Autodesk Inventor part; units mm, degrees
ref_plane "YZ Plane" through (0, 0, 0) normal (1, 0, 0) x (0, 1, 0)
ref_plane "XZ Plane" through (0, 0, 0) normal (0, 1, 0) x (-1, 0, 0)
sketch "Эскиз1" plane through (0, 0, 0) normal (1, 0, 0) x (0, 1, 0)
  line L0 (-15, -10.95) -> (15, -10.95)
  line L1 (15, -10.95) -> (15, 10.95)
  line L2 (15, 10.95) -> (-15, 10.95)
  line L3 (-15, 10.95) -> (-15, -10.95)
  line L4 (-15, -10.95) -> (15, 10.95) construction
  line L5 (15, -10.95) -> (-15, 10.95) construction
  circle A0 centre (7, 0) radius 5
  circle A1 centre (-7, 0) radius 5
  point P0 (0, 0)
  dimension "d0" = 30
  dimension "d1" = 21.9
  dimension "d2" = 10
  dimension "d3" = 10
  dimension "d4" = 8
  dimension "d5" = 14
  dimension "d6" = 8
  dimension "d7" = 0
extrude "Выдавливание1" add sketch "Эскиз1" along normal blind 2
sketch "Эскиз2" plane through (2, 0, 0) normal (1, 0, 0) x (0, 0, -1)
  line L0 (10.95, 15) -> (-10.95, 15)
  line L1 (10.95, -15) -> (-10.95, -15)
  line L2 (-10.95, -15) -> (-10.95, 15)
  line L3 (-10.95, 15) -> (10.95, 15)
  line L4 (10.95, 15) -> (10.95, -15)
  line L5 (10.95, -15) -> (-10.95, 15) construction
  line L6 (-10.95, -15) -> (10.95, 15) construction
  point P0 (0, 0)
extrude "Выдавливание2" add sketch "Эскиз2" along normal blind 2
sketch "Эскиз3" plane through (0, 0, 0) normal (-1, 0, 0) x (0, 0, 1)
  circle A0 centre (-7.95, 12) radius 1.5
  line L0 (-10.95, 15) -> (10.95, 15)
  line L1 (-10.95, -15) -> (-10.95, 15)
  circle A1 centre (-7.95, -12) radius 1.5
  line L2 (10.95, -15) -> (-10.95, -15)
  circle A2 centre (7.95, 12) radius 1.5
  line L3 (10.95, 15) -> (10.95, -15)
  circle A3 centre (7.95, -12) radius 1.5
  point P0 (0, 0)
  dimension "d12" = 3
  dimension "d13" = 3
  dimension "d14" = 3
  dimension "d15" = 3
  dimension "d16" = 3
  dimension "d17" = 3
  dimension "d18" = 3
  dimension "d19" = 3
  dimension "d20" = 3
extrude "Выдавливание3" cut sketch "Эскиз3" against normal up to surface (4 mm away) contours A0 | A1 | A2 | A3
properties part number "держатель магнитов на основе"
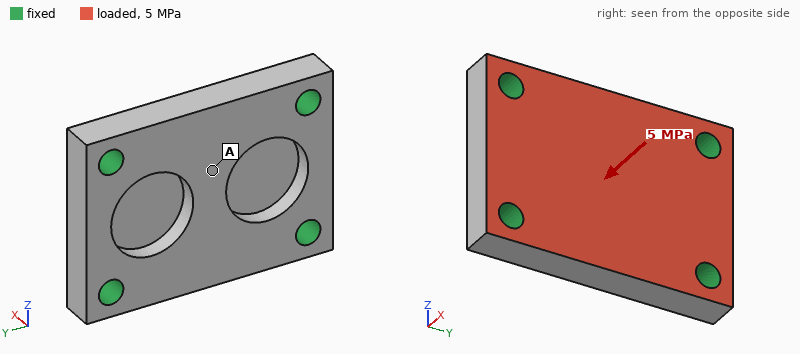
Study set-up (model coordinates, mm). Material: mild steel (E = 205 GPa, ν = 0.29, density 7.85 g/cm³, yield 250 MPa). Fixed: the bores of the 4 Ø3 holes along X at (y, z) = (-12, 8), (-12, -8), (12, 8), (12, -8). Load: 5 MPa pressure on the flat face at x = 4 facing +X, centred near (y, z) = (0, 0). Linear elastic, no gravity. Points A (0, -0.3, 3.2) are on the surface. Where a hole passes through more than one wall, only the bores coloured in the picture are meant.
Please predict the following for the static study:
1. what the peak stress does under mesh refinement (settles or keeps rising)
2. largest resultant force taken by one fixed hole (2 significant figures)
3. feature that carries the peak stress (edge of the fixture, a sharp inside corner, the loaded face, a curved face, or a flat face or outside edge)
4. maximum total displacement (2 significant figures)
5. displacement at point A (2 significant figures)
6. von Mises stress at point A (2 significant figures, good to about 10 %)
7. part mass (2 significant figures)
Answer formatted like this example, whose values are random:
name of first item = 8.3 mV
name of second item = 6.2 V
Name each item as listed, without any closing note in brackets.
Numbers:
what the peak stress does under mesh refinement = keeps rising
largest resultant force taken by one fixed hole = 800 N
feature that carries the peak stress = edge of the fixture
maximum total displacement = 7.9 µm
displacement at point A = 7.3 µm
von Mises stress at point A = 34 MPa
part mass = 17 g
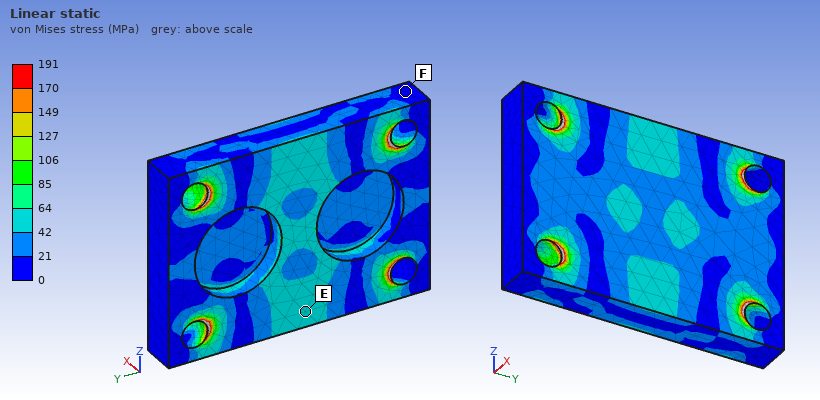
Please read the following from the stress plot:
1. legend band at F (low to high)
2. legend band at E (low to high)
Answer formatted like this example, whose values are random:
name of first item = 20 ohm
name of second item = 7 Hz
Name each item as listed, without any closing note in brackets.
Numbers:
legend band at F = 0 to 21 MPa
legend band at E = 42 to 64 MPa
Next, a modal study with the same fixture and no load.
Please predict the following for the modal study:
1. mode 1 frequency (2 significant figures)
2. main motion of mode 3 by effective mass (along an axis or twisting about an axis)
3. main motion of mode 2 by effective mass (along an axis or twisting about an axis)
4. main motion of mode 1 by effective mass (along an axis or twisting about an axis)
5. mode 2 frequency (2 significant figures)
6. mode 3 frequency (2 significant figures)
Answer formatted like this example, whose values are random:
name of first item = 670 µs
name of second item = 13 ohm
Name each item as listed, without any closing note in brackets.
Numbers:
mode 1 frequency = 29 kHz
main motion of mode 3 by effective mass = along Z
main motion of mode 2 by effective mass = twisting about Y
main motion of mode 1 by effective mass = along X
mode 2 frequency = 39 kHz
mode 3 frequency = 54 kHz
